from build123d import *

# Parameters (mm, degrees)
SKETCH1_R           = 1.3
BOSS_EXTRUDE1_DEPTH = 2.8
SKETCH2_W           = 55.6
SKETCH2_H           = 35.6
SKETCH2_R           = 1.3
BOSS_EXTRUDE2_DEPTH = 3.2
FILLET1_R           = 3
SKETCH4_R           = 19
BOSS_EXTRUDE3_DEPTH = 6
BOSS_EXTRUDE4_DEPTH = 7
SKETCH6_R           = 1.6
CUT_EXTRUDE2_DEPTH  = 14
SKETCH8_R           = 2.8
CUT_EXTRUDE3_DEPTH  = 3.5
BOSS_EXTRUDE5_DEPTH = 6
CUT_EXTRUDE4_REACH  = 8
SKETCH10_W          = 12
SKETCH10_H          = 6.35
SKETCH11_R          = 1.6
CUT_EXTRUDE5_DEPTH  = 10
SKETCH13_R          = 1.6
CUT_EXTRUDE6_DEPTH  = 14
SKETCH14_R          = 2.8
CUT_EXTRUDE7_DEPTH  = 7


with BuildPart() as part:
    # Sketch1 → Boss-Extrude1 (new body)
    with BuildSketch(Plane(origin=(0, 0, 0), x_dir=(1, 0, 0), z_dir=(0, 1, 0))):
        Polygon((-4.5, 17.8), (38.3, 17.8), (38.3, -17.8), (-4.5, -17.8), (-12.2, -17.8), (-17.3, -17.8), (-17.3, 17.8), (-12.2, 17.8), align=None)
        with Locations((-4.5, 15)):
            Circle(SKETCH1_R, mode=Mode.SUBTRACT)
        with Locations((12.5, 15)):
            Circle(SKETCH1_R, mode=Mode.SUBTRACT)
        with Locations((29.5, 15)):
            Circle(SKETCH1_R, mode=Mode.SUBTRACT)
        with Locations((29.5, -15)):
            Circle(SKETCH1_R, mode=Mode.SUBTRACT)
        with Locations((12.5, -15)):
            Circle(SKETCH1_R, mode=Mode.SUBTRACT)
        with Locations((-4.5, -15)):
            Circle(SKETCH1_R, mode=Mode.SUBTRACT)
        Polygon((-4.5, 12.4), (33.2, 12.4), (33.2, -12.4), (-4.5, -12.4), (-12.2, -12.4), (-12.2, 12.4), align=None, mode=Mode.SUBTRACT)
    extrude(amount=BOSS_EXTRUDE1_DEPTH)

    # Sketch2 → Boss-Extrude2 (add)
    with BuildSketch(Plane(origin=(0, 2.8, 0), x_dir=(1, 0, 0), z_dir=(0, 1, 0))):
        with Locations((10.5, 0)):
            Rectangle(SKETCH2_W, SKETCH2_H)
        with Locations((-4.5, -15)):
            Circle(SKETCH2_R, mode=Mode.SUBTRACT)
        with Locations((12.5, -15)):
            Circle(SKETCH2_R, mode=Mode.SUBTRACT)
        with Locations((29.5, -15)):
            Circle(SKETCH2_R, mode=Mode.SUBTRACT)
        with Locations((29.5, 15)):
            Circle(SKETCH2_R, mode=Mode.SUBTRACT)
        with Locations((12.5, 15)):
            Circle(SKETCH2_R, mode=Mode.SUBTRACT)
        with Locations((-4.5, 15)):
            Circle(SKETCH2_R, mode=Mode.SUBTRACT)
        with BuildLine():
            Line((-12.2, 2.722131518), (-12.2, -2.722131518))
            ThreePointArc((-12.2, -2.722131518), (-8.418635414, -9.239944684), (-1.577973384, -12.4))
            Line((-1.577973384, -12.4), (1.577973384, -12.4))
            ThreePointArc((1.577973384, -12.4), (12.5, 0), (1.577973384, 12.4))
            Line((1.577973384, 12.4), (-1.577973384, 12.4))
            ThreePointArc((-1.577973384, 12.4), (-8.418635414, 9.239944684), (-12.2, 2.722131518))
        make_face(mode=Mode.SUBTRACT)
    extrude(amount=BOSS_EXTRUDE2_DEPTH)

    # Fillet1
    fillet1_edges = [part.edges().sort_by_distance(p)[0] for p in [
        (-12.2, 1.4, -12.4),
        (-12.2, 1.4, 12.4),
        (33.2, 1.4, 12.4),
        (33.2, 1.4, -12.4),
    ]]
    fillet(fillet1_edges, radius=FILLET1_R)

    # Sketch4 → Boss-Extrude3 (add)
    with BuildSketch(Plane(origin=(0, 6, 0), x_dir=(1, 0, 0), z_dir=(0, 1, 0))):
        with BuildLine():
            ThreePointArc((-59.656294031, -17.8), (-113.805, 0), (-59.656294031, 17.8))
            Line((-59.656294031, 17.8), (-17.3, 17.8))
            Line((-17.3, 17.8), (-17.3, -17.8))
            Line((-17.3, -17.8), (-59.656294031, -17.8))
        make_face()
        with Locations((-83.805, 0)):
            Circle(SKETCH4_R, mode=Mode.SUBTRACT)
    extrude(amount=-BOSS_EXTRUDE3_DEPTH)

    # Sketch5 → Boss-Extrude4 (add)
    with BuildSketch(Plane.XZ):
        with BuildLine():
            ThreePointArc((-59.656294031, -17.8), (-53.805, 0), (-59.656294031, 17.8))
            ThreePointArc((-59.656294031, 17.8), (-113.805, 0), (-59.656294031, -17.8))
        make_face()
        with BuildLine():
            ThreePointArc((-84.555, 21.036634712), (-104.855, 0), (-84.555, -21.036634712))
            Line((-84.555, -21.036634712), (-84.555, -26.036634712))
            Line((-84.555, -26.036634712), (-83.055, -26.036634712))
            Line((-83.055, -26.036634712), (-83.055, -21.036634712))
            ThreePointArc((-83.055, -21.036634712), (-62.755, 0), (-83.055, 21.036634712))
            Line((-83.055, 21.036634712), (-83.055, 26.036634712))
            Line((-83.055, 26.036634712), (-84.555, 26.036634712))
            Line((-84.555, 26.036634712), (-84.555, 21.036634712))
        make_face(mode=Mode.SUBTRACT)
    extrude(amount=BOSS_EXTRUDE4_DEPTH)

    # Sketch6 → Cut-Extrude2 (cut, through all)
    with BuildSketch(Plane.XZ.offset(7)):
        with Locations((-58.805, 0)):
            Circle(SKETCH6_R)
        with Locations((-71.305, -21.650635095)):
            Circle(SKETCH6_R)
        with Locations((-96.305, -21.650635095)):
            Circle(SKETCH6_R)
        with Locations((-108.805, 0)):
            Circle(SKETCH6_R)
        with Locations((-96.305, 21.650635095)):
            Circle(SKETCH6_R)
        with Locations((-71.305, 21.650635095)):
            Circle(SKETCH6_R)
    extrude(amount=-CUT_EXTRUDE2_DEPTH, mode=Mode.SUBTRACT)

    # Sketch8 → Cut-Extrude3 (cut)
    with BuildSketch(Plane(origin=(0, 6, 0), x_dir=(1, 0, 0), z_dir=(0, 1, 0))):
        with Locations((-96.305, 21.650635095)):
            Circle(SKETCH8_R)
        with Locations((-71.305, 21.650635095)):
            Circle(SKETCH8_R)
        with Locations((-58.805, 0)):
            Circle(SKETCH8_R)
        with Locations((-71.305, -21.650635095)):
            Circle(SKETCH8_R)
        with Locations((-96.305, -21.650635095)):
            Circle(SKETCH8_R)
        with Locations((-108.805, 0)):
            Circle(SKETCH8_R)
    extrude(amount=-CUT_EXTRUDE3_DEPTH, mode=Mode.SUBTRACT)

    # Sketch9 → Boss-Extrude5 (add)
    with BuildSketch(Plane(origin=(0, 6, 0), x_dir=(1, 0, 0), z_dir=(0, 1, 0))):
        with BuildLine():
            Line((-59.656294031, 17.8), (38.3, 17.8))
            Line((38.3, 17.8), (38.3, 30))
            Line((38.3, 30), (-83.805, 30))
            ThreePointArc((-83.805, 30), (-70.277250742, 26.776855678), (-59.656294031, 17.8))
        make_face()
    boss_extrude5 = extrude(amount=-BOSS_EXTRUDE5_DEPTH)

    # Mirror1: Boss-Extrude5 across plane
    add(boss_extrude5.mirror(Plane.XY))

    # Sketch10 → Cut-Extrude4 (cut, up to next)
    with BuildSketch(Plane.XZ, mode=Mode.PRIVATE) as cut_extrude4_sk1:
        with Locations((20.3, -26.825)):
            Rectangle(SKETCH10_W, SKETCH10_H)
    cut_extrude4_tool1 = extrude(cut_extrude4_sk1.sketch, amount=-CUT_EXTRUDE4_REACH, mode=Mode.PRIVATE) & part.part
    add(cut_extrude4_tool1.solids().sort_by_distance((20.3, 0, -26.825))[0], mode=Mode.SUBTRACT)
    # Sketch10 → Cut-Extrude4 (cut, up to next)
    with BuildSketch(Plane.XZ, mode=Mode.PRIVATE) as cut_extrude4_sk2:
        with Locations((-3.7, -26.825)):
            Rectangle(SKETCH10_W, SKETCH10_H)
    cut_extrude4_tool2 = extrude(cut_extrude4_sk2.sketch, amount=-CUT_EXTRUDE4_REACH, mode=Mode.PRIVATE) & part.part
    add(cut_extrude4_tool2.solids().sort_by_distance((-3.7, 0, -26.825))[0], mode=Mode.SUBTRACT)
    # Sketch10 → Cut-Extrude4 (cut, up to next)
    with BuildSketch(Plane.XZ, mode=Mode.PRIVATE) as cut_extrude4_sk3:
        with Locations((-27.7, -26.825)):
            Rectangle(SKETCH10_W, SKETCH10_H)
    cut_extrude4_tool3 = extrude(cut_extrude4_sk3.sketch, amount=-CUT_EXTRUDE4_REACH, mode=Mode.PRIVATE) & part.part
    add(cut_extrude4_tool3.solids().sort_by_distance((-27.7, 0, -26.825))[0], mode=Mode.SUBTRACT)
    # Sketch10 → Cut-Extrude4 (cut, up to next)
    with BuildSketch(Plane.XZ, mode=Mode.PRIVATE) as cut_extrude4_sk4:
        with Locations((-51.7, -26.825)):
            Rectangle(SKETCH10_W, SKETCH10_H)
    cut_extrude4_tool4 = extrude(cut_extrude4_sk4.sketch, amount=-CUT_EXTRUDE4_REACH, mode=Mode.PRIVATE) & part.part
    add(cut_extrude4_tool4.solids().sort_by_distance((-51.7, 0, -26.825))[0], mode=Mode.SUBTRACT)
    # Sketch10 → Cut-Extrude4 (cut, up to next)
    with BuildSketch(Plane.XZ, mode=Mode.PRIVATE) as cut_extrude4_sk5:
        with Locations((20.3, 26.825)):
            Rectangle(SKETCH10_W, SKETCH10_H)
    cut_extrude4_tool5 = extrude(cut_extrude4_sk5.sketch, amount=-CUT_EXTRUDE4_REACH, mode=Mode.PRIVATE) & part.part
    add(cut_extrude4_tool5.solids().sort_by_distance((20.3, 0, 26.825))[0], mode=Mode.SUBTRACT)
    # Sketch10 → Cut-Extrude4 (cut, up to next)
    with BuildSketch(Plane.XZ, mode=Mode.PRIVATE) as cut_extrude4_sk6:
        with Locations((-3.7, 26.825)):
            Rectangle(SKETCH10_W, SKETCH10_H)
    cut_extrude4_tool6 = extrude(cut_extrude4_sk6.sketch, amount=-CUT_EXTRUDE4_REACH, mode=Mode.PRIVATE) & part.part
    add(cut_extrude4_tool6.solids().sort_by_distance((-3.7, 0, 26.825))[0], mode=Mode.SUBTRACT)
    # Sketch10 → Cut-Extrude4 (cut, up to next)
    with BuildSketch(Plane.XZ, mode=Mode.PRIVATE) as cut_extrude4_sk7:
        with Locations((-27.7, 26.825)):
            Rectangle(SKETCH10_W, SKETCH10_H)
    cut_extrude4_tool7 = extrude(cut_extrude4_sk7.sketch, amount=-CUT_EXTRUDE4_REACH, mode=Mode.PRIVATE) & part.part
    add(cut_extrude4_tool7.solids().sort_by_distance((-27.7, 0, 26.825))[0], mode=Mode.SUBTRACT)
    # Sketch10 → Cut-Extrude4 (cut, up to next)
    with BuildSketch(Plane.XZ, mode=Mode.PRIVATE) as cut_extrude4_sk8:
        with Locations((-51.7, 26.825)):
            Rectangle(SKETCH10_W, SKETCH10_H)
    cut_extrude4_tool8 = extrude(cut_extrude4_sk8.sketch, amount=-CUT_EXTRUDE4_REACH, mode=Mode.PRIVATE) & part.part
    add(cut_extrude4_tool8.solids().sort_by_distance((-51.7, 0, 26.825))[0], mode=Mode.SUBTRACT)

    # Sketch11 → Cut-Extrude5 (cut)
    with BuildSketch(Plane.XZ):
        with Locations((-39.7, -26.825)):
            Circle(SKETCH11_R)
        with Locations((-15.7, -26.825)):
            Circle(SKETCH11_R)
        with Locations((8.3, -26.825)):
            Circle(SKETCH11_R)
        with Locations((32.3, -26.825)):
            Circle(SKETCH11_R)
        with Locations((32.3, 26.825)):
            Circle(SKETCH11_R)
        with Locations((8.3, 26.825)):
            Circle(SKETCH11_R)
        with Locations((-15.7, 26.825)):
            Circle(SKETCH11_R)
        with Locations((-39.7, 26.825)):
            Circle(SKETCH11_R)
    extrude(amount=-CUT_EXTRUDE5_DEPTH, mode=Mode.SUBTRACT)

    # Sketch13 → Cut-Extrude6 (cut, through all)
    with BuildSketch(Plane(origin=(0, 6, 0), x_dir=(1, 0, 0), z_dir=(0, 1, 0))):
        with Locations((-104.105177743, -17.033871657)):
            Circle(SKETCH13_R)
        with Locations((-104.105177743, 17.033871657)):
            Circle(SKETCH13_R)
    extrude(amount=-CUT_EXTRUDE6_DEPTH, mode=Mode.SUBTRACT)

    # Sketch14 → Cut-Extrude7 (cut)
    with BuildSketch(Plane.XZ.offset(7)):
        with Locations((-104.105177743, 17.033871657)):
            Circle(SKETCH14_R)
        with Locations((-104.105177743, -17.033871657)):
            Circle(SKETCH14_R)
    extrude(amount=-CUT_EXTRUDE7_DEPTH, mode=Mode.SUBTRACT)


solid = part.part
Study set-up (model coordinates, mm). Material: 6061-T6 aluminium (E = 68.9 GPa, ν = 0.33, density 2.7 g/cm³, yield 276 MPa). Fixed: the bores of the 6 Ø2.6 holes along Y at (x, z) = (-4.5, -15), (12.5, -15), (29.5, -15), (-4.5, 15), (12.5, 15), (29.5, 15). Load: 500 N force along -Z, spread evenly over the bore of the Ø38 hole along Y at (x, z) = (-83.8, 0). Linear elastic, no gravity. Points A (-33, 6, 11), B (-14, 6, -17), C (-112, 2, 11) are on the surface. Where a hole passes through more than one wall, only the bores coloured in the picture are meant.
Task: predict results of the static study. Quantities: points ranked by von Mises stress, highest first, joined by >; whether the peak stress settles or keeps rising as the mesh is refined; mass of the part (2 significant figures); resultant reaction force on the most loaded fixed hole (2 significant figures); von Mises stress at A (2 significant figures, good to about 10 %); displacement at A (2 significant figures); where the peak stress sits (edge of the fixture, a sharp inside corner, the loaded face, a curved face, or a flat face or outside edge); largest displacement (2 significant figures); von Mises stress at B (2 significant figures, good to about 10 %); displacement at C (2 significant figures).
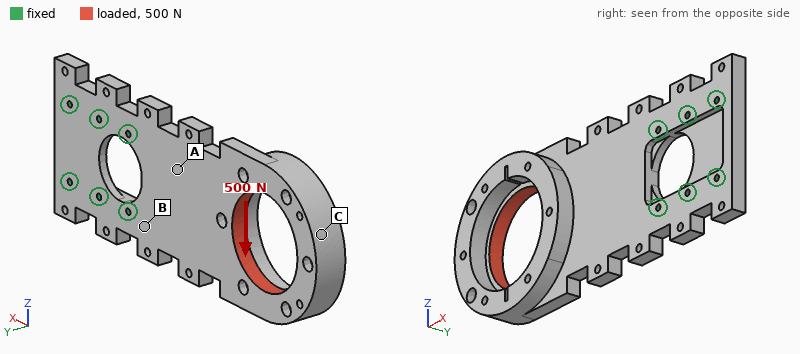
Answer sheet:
B > A > C
keeps rising
120 g
930 N
6.5 MPa
9.7 µm
edge of the fixture
64 µm
12 MPa
62 µm
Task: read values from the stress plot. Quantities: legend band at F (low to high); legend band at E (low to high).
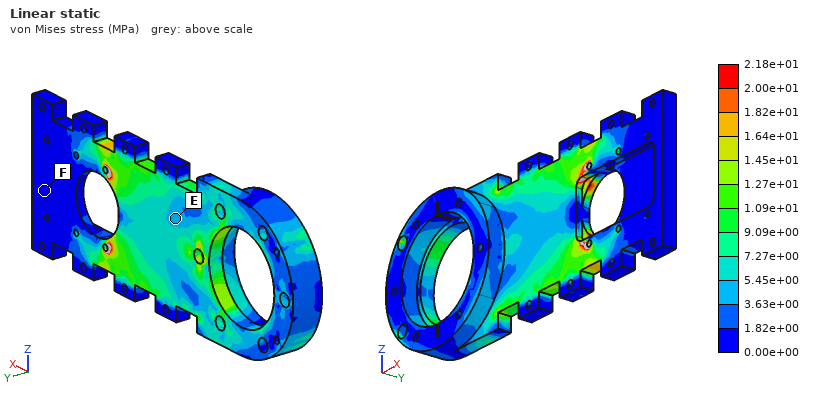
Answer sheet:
0.00e+00 to 1.82e+00 MPa
3.63e+00 to 5.45e+00 MPa
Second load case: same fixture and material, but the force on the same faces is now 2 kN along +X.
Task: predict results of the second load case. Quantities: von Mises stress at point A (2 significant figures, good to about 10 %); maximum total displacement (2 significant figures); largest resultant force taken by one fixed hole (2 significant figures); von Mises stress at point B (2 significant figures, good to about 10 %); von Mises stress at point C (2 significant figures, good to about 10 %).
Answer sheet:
6.2 MPa
25 µm
870 N
10 MPa
7.8 MPa
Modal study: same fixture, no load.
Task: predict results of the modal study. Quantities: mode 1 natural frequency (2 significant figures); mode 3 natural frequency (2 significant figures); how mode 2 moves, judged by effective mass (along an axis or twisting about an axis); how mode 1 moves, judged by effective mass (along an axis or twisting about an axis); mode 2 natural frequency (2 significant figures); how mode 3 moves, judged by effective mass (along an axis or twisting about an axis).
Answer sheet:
340 Hz
2200 Hz
twisting about X
along Y
1400 Hz
along Z
